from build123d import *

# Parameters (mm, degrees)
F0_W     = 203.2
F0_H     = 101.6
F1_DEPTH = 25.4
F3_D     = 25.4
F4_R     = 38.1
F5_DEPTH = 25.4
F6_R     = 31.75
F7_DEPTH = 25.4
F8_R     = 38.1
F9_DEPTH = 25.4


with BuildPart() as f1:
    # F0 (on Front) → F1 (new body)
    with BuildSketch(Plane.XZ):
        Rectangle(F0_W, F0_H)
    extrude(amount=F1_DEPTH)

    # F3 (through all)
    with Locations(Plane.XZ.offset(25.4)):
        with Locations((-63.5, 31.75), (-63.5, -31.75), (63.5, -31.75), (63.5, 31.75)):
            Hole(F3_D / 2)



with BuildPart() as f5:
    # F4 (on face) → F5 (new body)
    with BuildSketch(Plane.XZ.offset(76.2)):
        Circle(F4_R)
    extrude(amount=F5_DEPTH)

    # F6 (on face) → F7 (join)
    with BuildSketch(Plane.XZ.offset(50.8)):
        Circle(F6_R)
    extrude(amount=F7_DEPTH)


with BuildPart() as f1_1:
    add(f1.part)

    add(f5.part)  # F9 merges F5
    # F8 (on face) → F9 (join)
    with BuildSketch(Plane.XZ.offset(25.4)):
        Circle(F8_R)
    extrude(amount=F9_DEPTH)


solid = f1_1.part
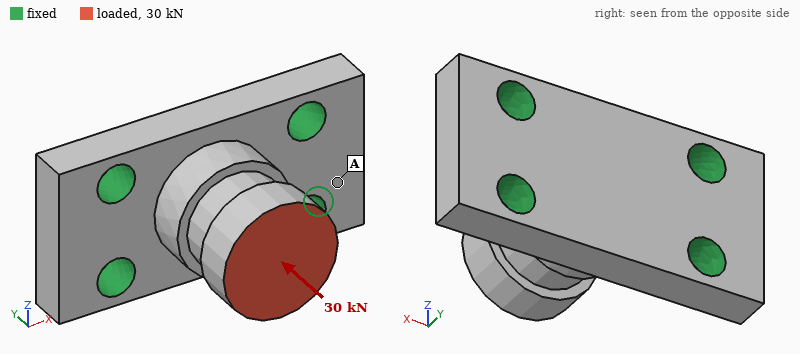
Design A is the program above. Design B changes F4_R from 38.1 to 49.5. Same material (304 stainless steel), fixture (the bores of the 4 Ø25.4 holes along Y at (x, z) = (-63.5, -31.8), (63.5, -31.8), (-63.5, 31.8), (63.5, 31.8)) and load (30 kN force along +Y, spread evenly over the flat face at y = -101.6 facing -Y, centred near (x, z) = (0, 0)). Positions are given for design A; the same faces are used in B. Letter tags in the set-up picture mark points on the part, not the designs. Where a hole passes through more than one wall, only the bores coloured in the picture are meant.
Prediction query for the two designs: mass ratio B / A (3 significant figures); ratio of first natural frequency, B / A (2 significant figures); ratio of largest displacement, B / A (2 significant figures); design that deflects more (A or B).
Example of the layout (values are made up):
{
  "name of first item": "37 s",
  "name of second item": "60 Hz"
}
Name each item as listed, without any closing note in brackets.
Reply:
{
  "mass ratio B / A": "1.10",
  "ratio of first natural frequency, B / A": "0.80",
  "ratio of largest displacement, B / A": "1.1",
  "design that deflects more": "B"
}
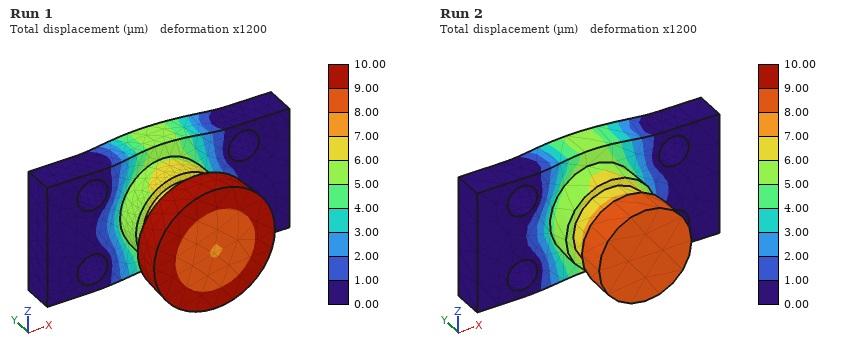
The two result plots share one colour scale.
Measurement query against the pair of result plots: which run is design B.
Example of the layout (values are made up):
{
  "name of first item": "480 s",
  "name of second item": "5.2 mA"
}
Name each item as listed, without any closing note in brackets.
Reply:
{
  "which run is design B": "Run 1"
}
